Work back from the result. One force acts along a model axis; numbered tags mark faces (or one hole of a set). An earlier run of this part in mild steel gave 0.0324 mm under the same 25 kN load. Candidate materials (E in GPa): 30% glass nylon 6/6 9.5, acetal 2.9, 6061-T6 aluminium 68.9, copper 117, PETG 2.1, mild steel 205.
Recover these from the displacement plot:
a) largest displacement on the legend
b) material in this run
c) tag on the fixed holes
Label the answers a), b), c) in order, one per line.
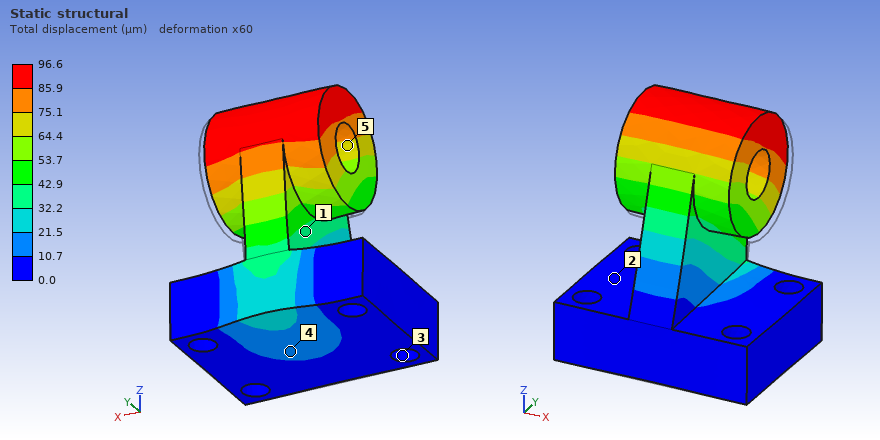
a) 96.6 µm
b) 6061-T6 aluminium
c) 3
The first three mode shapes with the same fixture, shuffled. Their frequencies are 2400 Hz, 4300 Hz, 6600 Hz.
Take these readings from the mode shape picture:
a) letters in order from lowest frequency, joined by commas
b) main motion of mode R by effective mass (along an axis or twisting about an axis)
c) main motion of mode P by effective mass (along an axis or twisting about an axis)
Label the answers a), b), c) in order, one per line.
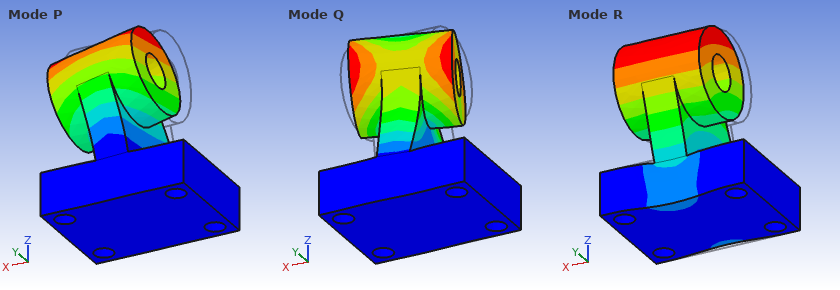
a) P, R, Q
b) along Y
c) along X
